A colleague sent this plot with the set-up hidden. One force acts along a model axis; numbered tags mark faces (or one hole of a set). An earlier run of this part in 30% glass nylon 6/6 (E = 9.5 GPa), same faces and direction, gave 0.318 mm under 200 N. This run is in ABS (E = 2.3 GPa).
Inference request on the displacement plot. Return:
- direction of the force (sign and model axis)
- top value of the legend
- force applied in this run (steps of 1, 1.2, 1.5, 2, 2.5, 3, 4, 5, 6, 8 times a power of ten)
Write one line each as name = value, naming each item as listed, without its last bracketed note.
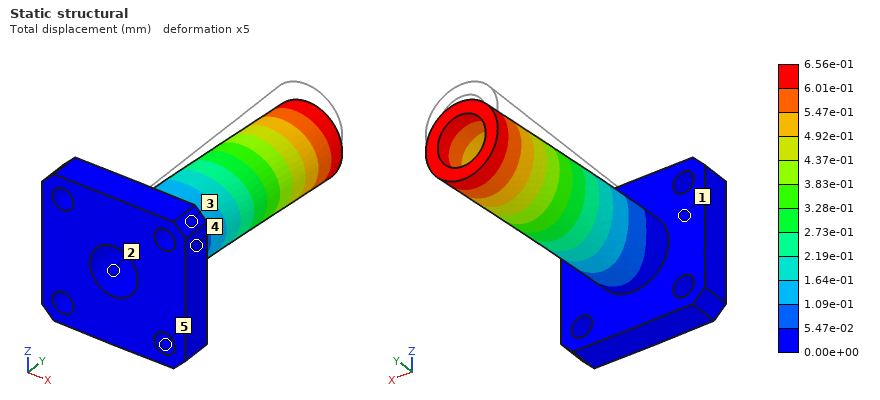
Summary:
direction of the force = -Z
top value of the legend = 6.56e-01 mm
force applied in this run = 100 N
